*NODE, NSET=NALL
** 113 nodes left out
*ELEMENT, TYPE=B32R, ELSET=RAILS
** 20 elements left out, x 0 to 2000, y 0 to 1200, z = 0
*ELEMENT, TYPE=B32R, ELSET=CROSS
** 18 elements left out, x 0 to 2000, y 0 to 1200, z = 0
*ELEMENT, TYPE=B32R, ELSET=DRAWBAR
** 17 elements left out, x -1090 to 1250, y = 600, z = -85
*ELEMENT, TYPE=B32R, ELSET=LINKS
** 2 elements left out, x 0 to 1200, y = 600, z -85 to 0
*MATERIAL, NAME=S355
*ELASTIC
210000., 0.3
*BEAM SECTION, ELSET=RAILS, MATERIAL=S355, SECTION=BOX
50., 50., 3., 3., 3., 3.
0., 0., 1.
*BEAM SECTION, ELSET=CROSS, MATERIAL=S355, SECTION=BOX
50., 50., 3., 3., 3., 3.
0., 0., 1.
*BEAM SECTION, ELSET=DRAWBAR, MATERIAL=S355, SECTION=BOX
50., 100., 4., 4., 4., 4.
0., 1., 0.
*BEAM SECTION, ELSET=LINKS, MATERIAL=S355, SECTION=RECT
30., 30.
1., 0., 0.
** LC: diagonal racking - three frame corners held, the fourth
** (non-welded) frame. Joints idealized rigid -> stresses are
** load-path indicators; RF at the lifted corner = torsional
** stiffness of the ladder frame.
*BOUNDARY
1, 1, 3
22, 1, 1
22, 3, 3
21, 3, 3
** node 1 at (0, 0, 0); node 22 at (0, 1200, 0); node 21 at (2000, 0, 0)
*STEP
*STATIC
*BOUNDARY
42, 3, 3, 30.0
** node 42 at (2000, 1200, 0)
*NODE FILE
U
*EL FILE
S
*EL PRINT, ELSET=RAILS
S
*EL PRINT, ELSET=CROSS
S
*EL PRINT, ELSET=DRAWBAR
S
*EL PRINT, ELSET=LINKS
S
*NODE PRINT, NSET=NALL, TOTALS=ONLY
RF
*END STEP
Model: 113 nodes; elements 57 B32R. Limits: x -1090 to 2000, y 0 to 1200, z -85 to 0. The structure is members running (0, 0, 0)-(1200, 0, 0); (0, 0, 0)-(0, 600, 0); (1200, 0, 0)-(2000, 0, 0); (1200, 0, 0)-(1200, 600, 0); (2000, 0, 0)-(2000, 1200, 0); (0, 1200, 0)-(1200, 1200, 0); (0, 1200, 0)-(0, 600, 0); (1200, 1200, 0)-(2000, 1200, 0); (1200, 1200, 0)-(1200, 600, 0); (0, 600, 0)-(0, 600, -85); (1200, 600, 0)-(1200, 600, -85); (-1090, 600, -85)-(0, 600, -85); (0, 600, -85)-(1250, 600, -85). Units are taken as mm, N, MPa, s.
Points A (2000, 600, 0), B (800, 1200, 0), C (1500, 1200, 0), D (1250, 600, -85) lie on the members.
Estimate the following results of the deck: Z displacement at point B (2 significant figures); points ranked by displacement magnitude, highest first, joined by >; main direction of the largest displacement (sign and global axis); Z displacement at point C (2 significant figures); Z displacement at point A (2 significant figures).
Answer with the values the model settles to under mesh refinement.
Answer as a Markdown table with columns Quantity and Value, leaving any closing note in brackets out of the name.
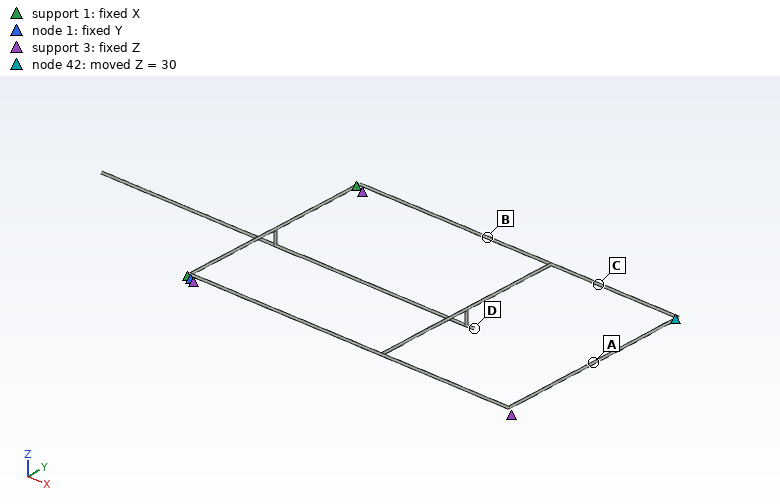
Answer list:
| Quantity | Value |
|---|---|
| Z displacement at point B | 12 mm |
| points ranked by displacement magnitude, highest first, joined by > | C > A > B > D |
| main direction of the largest displacement | +Z |
| Z displacement at point C | 23 mm |
| Z displacement at point A | 15 mm |
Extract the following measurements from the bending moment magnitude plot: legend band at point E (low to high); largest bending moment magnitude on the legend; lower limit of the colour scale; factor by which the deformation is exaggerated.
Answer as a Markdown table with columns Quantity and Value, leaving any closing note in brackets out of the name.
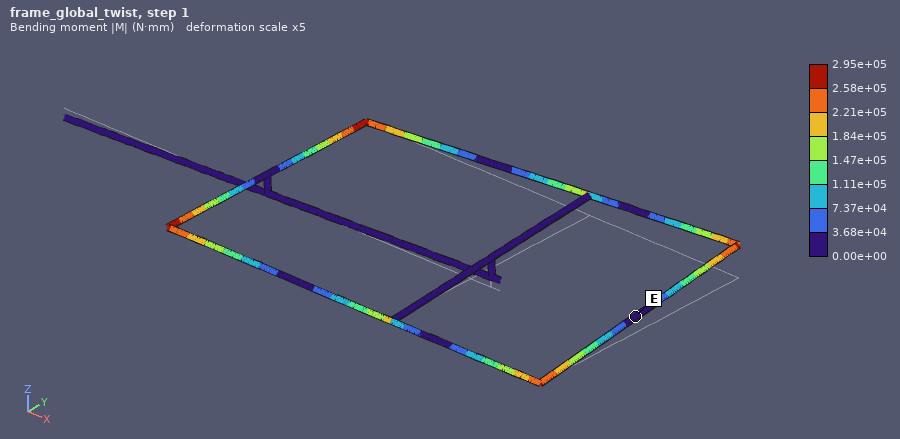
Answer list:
| Quantity | Value |
|---|---|
| legend band at point E | 0.00e+00 to 3.68e+04 N·mm |
| largest bending moment magnitude on the legend | 2.95e+05 N·mm |
| lower limit of the colour scale | 0.00e+00 N·mm |
| factor by which the deformation is exaggerated | 5 |
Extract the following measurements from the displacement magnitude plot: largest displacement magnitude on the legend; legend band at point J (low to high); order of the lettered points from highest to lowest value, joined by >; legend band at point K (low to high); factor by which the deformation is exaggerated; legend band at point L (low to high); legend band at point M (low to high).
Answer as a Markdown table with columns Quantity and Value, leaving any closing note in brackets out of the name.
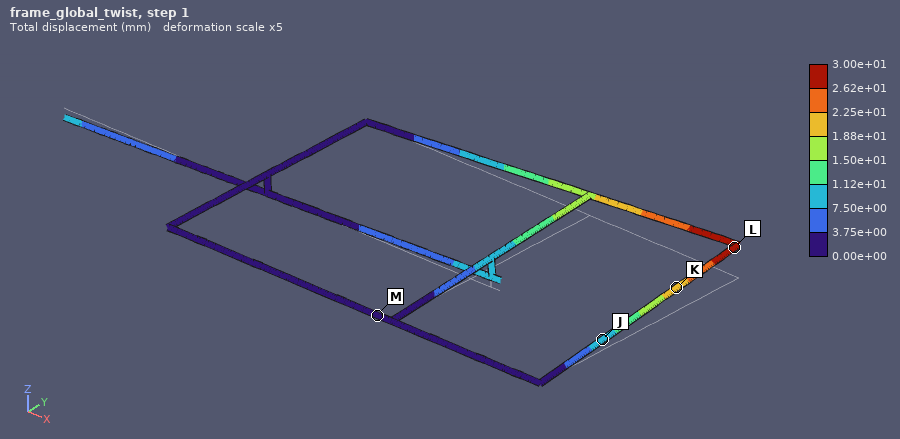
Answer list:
| Quantity | Value |
|---|---|
| largest displacement magnitude on the legend | 3.00e+01 mm |
| legend band at point J | 7.50e+00 to 1.12e+01 mm |
| order of the lettered points from highest to lowest value, joined by > | L > K > J > M |
| legend band at point K | 1.88e+01 to 2.25e+01 mm |
| factor by which the deformation is exaggerated | 5 |
| legend band at point L | 2.62e+01 to 3.00e+01 mm |
| legend band at point M | 0.00e+00 to 3.75e+00 mm |
